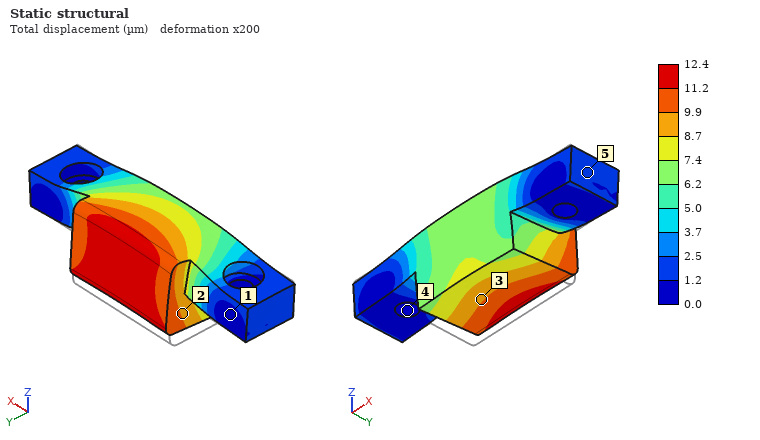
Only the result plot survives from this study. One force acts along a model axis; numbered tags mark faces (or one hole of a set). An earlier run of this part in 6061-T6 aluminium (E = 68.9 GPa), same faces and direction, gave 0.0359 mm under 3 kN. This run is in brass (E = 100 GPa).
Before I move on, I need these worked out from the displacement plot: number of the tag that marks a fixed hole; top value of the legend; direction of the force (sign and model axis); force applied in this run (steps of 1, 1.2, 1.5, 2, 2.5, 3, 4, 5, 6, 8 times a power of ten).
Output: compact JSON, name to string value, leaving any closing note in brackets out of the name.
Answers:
{"number of the tag that marks a fixed hole": "4", "top value of the legend": "12.4 µm", "direction of the force": "+Z", "force applied in this run": "1.5 kN"}
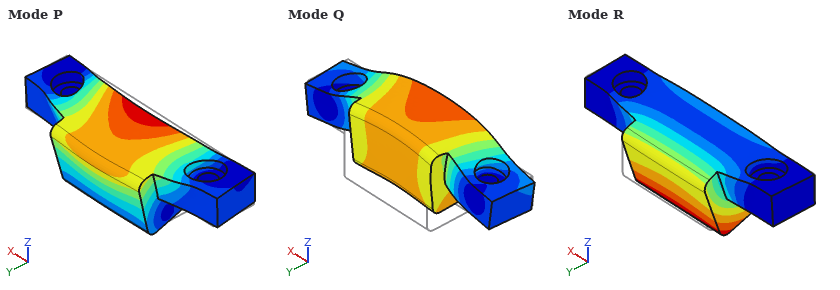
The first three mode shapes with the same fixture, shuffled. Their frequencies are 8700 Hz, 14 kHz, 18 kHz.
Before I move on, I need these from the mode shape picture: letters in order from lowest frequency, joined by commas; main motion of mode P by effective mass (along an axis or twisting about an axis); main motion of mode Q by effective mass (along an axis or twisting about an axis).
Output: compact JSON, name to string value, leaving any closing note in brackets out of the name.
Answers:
{"letters in order from lowest frequency, joined by commas": "R, Q, P", "main motion of mode P by effective mass": "along Y", "main motion of mode Q by effective mass": "along Z"}
